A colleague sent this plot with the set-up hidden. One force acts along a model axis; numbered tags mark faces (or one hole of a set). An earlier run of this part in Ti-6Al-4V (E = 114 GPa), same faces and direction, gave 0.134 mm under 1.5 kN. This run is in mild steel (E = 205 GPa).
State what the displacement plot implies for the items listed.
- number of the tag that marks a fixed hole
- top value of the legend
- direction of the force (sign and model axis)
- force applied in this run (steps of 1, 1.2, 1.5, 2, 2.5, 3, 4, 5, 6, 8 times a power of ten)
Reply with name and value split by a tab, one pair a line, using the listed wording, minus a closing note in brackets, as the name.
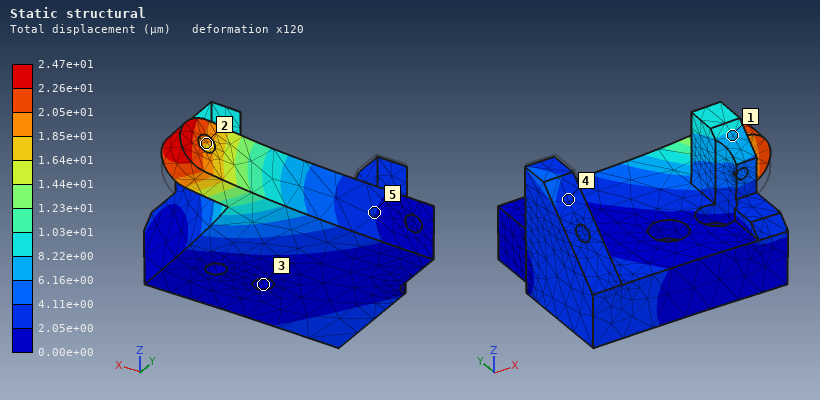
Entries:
number of the tag that marks a fixed hole	3
top value of the legend	2.47e+01 µm
direction of the force	+Z
force applied in this run	500 N
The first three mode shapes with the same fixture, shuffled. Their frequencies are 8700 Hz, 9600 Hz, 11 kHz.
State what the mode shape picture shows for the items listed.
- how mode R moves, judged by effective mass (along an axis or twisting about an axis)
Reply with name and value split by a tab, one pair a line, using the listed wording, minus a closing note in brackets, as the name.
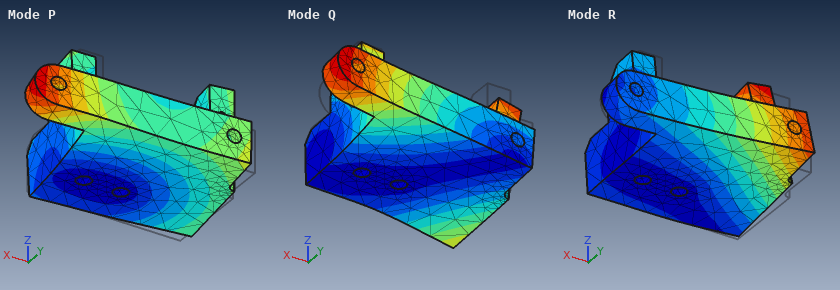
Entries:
how mode R moves, judged by effective mass	along Z
